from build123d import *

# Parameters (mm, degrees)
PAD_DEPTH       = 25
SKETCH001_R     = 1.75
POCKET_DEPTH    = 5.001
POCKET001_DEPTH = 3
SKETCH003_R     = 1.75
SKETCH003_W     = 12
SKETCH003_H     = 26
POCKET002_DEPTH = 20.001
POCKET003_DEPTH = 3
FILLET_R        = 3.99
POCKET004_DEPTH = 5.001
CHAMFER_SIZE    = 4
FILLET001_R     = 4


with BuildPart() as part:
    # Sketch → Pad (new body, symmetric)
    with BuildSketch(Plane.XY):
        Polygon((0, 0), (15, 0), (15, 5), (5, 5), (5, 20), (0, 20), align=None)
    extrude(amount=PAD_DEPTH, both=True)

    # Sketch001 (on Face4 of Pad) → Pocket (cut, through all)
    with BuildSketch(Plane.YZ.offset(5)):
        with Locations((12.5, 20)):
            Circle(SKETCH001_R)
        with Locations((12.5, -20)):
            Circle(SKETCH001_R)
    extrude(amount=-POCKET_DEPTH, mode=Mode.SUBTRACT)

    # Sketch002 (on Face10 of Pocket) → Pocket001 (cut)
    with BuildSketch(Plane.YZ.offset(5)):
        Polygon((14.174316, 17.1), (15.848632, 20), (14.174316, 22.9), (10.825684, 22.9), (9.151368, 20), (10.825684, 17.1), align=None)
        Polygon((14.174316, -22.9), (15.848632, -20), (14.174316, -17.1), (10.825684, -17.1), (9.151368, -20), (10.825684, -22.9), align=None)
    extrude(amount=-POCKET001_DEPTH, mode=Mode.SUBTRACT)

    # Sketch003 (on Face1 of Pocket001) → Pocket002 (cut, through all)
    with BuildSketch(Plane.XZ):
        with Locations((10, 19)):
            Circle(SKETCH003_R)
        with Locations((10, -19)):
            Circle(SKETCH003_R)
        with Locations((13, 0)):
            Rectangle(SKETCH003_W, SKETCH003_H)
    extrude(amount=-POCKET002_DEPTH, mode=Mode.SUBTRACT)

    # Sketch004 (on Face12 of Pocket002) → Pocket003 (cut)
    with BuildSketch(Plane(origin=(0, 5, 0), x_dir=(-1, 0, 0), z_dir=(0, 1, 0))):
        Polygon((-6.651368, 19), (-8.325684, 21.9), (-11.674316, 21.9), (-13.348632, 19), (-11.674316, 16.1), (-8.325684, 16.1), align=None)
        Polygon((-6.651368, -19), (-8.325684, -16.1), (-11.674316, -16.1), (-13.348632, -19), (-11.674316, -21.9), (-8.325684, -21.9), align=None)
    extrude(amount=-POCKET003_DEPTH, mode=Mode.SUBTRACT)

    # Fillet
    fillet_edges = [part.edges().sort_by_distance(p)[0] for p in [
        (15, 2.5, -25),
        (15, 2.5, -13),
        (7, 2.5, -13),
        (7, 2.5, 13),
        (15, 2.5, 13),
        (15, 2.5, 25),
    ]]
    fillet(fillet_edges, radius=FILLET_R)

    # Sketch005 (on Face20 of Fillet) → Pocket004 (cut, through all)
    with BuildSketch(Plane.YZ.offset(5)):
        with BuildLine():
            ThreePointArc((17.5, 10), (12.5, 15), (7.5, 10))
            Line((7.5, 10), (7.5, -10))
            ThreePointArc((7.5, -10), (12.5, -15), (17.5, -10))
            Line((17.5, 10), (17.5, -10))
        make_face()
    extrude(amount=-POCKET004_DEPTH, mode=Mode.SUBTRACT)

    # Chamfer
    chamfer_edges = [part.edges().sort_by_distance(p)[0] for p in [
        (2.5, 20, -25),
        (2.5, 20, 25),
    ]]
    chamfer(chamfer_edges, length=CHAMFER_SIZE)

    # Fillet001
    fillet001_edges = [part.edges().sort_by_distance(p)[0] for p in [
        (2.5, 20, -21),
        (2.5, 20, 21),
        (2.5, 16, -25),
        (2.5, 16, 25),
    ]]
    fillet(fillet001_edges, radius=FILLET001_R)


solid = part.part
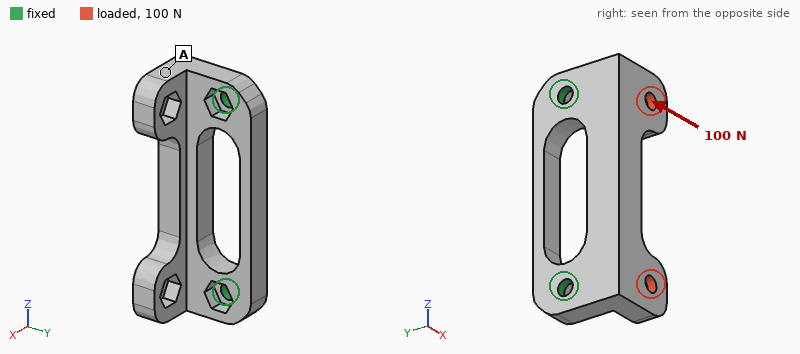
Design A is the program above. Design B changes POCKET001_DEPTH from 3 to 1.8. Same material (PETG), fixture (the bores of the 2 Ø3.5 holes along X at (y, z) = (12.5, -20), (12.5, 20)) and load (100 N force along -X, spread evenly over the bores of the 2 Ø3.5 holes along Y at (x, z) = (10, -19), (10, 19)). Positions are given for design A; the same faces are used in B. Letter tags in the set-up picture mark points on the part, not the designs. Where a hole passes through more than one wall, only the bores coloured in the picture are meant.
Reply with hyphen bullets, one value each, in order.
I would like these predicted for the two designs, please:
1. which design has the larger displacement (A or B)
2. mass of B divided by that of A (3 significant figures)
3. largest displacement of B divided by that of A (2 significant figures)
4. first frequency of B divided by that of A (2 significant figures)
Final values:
- A
- 1.01
- 0.60
- 1.3
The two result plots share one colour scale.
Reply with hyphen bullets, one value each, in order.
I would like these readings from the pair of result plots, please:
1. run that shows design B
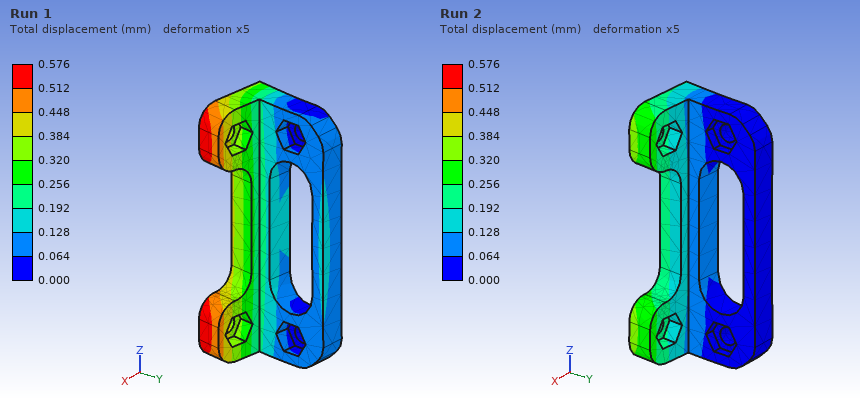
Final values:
- Run 2
